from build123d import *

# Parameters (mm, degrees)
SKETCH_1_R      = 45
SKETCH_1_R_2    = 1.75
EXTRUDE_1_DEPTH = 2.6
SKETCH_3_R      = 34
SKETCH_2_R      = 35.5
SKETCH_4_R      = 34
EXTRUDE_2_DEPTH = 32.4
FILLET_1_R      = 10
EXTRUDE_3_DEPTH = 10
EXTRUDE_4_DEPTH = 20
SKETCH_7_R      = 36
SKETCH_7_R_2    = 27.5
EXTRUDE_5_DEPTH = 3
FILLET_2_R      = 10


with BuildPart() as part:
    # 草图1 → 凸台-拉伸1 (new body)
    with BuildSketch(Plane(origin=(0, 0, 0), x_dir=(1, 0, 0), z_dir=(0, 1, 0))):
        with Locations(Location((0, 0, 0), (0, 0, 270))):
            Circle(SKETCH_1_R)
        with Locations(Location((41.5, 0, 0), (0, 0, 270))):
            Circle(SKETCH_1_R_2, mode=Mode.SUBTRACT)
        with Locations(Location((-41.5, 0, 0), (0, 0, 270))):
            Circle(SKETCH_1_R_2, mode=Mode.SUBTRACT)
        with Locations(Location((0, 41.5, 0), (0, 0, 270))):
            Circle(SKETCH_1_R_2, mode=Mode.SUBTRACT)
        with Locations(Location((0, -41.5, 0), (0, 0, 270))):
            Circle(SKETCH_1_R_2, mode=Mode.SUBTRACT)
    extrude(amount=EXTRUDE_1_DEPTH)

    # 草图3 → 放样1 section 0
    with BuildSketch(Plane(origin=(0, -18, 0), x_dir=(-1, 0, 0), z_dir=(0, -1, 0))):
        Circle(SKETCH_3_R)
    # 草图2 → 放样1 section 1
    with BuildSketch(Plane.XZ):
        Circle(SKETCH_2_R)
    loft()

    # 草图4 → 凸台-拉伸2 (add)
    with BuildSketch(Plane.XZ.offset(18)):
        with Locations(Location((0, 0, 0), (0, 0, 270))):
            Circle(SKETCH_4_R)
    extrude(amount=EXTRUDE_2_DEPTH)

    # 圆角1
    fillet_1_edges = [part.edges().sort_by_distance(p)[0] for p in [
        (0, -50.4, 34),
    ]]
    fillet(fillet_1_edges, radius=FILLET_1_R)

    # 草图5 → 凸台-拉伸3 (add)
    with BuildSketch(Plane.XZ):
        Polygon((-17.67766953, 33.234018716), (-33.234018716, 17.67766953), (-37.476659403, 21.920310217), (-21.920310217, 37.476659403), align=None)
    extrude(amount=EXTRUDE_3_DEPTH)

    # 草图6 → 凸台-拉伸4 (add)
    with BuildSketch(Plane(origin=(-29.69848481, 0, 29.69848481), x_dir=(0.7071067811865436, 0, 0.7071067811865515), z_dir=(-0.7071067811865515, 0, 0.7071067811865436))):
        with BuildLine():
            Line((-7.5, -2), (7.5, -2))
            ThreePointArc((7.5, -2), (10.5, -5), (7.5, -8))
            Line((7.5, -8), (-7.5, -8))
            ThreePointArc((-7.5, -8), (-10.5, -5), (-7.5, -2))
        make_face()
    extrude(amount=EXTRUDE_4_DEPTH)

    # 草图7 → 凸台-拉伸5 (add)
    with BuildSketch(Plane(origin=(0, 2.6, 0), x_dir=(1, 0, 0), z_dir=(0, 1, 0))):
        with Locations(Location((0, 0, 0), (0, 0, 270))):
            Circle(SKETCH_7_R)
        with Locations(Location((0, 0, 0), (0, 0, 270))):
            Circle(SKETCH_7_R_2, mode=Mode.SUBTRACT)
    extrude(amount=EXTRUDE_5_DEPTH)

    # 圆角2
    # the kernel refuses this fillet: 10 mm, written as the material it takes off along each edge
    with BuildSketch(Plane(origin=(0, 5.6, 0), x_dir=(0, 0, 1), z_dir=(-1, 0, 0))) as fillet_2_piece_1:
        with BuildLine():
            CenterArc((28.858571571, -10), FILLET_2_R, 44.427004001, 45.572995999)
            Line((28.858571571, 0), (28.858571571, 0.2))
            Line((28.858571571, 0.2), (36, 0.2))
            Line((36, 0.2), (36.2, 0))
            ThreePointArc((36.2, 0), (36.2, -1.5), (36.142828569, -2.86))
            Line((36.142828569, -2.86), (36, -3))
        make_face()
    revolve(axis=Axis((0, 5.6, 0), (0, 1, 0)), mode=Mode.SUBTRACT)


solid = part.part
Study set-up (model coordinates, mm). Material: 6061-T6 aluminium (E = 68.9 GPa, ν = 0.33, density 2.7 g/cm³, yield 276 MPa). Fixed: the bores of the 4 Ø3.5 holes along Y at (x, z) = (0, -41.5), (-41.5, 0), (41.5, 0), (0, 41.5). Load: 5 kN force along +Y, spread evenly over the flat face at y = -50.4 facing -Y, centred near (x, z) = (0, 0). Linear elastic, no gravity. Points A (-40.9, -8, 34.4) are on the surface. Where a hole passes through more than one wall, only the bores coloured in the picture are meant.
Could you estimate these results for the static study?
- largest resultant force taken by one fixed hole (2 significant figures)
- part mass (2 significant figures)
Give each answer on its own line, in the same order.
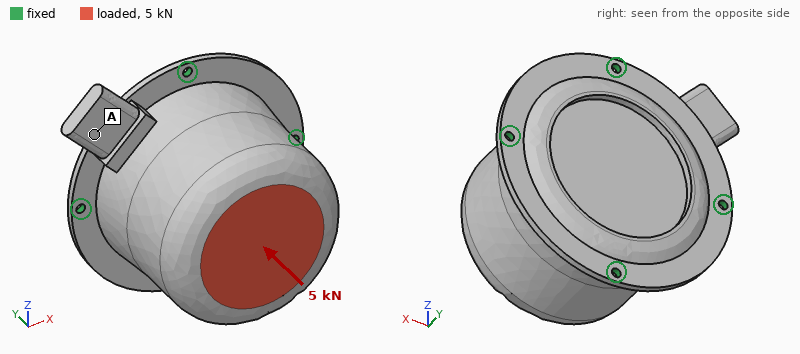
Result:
1.3 kN
550 g
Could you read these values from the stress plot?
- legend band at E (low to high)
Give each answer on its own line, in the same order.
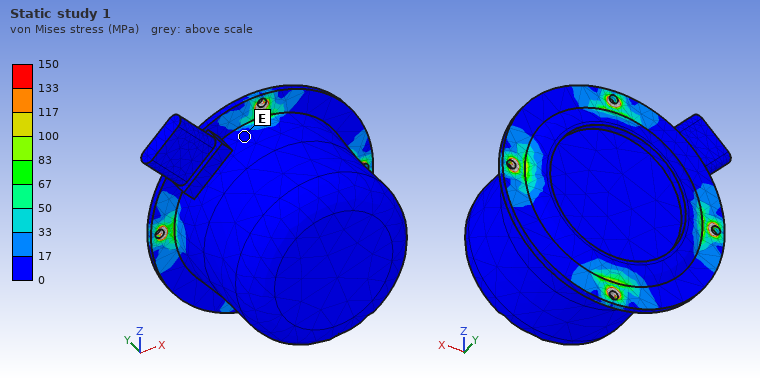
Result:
0 to 17 MPa
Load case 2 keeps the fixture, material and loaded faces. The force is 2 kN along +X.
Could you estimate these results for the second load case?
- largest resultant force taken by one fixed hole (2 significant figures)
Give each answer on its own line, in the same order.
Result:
1.5 kN
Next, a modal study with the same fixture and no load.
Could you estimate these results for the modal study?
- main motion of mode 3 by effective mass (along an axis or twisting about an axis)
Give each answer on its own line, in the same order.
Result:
along Y
